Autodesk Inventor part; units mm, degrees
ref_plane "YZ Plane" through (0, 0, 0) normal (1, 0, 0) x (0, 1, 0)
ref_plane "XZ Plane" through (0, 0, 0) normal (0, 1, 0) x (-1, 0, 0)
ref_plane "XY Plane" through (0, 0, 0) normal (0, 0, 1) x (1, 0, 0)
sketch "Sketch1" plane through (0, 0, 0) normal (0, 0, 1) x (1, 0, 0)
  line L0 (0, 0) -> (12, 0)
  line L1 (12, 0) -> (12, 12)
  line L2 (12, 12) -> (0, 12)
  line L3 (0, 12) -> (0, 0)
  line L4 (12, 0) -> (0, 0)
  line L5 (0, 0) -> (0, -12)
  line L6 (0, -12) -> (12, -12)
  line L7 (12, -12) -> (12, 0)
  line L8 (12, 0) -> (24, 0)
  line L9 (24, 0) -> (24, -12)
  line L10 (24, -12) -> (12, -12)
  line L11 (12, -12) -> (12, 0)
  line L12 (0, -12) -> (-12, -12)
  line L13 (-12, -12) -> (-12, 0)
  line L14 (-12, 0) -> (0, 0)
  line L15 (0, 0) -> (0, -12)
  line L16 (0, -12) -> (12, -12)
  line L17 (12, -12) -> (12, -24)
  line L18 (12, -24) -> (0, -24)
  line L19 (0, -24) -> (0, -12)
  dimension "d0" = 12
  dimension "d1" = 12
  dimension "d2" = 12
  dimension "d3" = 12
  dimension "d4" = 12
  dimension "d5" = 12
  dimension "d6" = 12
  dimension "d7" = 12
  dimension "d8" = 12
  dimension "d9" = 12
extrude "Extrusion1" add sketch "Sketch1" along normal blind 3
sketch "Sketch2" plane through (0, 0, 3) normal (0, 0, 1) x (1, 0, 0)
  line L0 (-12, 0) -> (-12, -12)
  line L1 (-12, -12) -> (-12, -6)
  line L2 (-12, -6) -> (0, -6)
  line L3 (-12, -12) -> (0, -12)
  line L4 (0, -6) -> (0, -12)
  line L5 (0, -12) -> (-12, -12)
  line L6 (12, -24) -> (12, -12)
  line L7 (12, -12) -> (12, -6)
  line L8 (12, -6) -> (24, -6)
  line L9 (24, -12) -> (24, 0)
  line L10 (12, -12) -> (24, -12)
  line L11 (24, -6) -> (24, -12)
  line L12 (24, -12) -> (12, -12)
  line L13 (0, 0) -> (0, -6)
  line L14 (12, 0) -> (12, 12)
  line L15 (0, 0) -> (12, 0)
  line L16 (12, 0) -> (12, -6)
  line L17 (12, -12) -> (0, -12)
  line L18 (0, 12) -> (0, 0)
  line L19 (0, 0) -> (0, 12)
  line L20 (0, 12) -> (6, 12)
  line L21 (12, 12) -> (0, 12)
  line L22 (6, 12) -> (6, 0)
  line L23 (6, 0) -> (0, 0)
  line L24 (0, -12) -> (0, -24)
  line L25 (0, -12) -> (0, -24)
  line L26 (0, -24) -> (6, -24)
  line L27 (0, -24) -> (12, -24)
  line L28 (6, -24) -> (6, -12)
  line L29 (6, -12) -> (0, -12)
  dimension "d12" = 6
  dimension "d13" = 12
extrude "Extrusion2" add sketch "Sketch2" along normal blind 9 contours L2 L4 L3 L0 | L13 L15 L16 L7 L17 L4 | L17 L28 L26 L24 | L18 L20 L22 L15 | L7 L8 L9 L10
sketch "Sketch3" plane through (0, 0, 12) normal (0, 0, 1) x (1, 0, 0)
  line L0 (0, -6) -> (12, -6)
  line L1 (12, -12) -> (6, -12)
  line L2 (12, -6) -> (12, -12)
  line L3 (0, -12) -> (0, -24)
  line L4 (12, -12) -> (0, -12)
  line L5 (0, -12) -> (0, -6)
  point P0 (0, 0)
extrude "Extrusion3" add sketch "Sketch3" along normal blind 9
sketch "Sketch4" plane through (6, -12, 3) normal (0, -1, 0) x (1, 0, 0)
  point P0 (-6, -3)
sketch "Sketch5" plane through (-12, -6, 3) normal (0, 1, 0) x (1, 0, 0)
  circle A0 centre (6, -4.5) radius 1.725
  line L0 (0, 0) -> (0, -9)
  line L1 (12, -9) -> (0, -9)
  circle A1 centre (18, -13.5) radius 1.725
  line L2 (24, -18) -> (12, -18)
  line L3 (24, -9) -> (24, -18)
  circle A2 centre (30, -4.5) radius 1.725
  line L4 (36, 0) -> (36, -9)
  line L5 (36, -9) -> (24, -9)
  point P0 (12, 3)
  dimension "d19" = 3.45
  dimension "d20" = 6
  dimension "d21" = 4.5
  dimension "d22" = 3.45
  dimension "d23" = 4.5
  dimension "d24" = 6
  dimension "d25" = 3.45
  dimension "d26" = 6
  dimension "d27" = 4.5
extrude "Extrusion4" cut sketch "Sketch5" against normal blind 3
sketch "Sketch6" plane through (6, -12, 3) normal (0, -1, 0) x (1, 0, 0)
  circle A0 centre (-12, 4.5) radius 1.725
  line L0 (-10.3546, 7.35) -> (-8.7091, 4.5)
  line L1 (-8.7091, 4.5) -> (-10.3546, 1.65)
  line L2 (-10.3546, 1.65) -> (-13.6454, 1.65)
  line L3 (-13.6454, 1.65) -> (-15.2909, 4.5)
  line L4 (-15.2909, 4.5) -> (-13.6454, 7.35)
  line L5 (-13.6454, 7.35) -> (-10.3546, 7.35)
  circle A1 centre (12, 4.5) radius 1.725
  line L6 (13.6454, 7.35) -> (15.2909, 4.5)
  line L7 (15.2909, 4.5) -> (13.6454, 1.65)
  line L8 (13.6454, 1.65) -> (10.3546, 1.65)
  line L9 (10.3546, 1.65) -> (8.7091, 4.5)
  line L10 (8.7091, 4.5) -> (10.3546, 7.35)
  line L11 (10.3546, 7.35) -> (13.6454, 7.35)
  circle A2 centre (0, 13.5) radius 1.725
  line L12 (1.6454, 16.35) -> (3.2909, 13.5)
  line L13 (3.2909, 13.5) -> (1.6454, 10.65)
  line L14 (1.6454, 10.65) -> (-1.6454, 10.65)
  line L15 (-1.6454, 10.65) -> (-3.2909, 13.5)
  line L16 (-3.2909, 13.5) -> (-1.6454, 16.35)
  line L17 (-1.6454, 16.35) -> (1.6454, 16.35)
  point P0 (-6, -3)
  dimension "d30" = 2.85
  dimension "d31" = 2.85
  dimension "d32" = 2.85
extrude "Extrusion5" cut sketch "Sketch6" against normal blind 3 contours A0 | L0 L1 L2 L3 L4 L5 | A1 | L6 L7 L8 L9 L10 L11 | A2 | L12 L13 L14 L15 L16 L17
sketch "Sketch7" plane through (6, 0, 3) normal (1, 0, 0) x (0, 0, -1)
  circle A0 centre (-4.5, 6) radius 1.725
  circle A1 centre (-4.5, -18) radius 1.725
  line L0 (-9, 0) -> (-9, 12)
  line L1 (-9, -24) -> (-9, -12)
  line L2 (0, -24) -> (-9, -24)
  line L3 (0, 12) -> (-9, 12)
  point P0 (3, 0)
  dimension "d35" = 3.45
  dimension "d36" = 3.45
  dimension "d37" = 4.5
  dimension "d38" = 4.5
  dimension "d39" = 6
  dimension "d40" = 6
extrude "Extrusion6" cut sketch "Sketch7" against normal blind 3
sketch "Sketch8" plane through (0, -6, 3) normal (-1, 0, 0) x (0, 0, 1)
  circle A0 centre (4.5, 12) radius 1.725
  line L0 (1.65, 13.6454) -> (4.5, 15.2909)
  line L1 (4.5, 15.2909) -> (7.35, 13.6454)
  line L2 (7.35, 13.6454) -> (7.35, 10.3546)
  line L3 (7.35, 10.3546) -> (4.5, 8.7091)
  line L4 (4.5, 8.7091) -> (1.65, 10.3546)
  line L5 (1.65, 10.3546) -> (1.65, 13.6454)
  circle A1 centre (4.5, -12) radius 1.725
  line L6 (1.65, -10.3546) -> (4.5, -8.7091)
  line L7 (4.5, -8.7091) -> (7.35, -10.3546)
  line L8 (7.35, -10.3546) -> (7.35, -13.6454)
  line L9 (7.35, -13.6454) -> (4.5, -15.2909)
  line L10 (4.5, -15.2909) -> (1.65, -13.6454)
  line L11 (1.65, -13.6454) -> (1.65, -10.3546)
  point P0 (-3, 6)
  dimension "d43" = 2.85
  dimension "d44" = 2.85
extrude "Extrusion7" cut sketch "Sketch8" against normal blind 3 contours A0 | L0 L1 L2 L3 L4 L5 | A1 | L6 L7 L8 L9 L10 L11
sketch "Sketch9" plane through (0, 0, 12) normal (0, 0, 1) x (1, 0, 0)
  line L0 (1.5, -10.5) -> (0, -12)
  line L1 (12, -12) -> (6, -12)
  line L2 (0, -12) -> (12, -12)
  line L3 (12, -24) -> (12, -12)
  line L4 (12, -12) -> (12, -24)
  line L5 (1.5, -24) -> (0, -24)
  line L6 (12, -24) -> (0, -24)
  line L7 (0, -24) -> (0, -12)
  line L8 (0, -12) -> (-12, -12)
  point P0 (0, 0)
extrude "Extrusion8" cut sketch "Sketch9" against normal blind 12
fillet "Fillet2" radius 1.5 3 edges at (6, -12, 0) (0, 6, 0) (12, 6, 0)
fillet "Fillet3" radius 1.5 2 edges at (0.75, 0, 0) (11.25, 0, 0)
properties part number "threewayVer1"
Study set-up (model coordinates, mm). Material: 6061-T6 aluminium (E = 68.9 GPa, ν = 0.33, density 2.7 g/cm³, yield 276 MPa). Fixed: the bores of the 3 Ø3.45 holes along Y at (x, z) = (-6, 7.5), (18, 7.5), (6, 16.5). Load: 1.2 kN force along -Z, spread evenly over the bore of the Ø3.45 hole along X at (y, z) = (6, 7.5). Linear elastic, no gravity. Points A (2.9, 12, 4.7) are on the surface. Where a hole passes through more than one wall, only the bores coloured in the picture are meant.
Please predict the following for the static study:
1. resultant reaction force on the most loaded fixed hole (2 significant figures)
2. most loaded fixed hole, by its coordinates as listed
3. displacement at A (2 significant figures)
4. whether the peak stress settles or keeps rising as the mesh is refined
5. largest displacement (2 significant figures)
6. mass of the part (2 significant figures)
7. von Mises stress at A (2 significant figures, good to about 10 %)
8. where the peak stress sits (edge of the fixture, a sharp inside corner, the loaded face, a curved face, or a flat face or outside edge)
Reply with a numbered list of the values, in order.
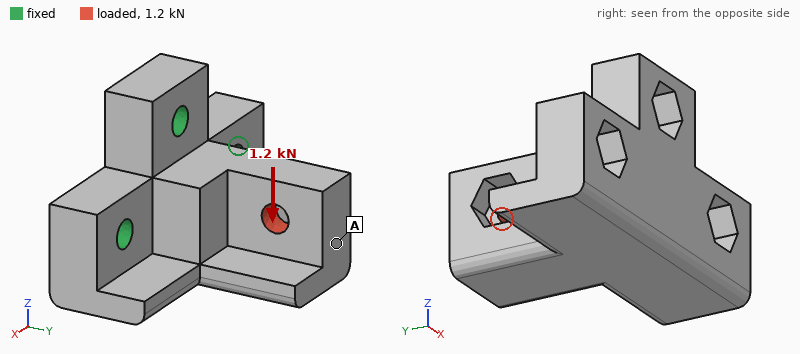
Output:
1. 1.4 kN
2. (6, 16.5)
3. 72 µm
4. keeps rising
5. 78 µm
6. 14 g
7. 15 MPa
8. edge of the fixture
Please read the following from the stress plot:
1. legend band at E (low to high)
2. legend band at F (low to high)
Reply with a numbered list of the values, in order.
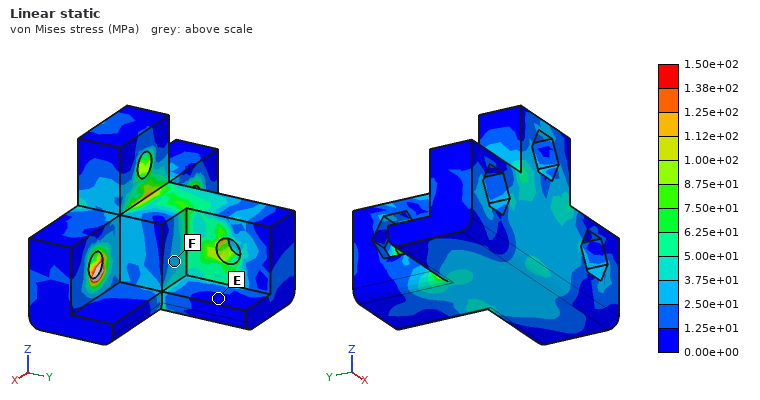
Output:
1. 0.00e+00 to 1.25e+01 MPa
2. 2.50e+01 to 3.75e+01 MPa
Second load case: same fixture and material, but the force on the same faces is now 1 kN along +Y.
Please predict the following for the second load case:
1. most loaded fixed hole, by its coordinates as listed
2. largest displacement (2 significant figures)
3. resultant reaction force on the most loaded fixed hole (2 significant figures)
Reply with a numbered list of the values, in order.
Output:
1. (-6, 7.5)
2. 10 µm
3. 440 N
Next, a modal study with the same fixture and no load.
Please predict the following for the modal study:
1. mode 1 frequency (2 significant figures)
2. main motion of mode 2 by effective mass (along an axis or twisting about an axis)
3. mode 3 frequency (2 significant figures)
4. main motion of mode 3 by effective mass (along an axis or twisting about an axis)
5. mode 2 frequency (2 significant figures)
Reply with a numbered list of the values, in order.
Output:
1. 12 kHz
2. along X
3. 27 kHz
4. along Y
5. 19 kHz
